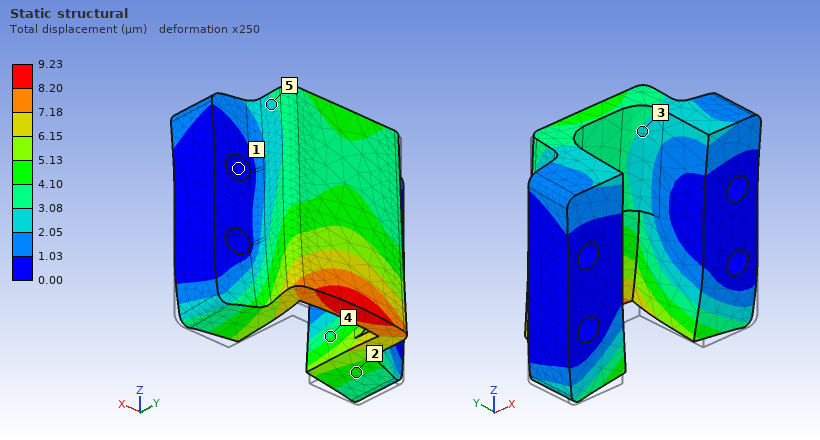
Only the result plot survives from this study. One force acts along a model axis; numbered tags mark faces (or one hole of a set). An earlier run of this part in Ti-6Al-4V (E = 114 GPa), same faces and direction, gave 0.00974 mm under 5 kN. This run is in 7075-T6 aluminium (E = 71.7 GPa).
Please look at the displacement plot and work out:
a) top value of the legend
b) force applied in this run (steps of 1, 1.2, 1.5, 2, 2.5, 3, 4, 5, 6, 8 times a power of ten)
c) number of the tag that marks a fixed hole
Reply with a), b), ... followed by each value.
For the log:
a) 9.23 µm
b) 3 kN
c) 1
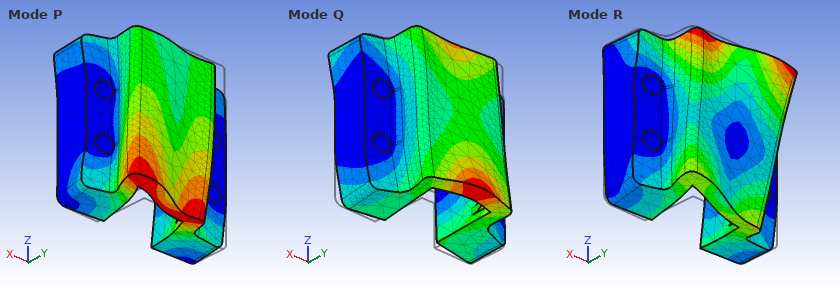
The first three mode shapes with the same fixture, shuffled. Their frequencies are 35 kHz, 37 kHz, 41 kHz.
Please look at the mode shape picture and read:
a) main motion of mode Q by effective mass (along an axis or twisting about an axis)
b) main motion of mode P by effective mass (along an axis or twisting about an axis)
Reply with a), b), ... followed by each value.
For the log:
a) along Z
b) along X
